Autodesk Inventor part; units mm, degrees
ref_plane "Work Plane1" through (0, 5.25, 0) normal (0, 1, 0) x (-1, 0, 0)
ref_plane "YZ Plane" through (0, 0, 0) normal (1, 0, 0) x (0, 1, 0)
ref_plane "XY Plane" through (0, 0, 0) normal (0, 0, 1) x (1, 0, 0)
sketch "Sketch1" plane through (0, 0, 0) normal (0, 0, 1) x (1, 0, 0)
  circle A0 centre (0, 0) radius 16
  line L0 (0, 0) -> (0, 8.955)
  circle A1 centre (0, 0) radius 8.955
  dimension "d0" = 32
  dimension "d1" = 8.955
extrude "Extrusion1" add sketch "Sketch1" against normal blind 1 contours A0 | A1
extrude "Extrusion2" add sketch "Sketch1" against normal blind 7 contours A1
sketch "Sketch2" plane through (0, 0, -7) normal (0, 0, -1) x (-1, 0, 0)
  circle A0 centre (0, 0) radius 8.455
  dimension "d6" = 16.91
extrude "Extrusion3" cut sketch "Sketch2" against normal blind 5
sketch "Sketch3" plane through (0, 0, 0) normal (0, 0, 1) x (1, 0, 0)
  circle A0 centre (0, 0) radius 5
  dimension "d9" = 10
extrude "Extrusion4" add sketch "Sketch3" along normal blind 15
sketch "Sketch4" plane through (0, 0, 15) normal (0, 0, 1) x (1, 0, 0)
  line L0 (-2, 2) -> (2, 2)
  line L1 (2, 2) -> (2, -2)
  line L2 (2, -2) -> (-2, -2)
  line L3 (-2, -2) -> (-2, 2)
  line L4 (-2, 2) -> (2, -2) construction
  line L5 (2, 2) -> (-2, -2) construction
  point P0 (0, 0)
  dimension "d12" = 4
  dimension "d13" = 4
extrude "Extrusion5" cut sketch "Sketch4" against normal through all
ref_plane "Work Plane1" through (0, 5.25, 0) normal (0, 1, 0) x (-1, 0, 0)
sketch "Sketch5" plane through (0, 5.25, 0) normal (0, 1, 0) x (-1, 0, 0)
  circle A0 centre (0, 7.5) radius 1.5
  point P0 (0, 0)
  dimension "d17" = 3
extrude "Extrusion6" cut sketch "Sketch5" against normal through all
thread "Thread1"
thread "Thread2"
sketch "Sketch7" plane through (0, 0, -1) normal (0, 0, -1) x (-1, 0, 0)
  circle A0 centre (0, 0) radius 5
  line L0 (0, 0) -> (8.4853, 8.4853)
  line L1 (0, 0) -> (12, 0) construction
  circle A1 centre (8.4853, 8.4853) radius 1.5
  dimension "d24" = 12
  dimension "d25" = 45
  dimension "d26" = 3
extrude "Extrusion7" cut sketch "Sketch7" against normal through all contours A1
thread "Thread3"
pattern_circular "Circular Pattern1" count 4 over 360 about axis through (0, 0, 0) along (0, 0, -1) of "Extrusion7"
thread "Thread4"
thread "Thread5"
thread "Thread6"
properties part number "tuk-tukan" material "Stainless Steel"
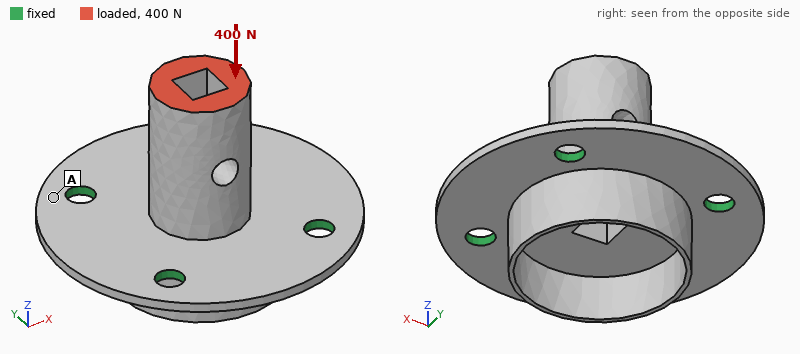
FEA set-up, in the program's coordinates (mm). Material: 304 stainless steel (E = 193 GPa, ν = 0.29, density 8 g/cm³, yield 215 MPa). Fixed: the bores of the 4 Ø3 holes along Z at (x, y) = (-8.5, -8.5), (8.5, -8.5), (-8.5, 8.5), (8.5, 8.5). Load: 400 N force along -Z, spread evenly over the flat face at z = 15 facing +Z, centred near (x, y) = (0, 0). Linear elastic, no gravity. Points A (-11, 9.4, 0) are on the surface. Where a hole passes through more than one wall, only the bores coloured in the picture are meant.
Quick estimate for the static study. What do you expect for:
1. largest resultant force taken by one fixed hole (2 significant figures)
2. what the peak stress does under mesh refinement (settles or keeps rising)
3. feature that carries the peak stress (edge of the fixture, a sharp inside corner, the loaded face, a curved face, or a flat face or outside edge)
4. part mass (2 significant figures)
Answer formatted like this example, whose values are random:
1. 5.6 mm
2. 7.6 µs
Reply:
1. 120 N
2. keeps rising
3. edge of the fixture
4. 16 g
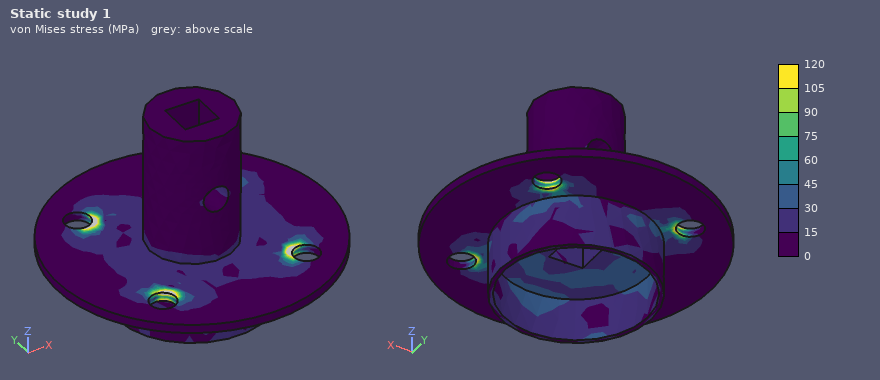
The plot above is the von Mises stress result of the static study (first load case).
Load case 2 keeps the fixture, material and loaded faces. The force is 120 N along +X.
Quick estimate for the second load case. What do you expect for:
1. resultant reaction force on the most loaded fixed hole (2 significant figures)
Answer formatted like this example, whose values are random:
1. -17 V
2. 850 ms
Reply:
1. 73 N
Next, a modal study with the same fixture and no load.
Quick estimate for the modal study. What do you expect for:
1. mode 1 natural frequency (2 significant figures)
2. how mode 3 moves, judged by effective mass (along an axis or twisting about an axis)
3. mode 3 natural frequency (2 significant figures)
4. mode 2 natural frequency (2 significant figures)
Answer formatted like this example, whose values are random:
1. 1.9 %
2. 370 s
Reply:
1. 9500 Hz
2. along Z
3. 14 kHz
4. 9600 Hz
